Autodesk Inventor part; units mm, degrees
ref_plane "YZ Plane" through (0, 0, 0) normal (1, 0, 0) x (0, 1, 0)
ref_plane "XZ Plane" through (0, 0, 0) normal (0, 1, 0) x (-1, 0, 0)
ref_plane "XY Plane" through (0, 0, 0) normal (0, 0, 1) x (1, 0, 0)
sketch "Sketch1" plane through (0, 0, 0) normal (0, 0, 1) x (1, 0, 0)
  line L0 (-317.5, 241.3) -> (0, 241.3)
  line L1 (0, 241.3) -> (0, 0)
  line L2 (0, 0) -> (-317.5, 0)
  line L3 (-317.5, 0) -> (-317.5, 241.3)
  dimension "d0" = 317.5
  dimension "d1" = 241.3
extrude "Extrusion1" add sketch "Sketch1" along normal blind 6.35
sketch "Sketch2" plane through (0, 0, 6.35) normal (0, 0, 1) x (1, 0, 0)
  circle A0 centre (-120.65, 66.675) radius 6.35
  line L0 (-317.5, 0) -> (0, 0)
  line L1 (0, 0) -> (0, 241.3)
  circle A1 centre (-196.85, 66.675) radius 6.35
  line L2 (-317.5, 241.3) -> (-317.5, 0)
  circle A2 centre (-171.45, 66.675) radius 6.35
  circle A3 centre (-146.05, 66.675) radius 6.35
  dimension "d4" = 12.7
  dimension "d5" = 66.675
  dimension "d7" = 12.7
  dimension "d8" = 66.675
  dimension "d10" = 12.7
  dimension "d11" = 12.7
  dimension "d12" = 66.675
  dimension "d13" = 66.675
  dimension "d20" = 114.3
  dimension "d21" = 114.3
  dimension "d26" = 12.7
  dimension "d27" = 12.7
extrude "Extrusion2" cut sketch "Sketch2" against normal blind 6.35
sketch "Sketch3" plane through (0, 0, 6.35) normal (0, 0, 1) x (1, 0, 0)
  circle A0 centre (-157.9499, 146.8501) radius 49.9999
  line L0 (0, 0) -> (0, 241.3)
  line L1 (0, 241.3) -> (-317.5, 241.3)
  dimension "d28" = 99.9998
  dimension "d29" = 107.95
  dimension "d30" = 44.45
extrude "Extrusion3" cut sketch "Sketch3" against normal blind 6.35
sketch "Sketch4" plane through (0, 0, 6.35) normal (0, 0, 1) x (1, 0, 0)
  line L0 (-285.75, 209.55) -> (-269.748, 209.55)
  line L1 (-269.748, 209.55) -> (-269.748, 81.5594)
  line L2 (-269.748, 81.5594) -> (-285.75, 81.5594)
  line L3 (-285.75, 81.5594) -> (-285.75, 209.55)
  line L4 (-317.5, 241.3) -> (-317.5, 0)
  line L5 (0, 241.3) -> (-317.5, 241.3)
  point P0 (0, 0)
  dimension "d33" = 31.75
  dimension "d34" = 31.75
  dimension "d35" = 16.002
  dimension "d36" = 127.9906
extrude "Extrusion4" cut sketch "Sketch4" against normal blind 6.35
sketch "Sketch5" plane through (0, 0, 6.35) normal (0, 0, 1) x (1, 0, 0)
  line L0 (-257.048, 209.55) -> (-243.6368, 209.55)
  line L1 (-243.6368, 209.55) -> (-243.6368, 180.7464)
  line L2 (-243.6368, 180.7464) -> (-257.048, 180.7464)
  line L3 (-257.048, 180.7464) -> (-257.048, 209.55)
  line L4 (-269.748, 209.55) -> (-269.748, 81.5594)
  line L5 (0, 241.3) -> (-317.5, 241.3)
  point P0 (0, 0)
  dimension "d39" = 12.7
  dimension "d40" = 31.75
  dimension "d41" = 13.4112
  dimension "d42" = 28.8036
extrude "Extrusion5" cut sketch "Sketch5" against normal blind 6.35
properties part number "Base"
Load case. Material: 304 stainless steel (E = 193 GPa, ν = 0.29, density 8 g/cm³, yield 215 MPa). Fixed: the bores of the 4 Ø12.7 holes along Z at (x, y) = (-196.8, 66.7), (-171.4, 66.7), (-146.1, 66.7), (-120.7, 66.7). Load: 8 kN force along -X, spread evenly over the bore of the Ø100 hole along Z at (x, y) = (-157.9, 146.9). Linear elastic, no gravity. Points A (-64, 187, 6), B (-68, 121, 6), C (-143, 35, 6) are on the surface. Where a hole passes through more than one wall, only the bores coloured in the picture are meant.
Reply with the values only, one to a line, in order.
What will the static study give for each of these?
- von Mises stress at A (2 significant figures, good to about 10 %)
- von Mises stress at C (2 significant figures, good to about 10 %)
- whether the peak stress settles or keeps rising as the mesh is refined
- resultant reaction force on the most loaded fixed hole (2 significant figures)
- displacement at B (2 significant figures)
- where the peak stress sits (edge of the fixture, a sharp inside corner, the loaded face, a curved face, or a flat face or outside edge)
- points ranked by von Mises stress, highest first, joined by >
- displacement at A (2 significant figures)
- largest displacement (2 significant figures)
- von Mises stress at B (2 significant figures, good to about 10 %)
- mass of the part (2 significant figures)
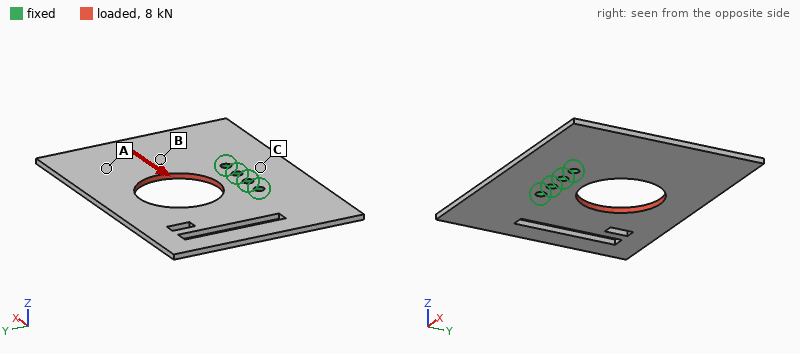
4.1 MPa
16 MPa
keeps rising
7.3 kN
25 µm
edge of the fixture
C > B > A
45 µm
67 µm
8.6 MPa
3.3 kg
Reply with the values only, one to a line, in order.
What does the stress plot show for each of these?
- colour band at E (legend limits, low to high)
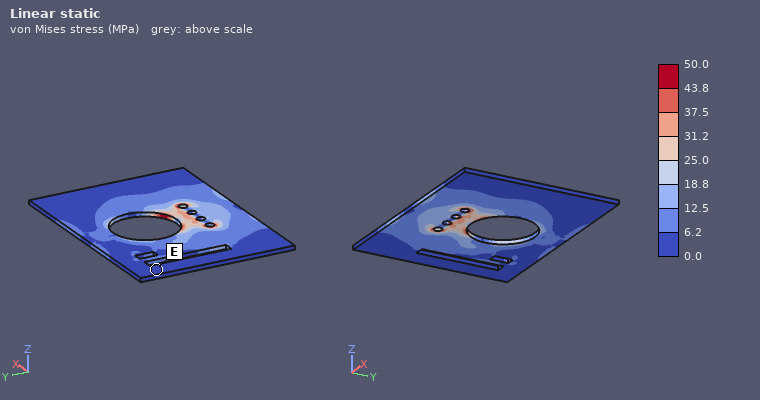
0.0 to 6.2 MPa
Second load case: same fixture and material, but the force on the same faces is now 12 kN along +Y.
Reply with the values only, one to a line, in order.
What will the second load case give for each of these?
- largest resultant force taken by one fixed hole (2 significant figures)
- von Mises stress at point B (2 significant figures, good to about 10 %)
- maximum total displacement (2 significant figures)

5.3 kN
6.2 MPa
18 µm
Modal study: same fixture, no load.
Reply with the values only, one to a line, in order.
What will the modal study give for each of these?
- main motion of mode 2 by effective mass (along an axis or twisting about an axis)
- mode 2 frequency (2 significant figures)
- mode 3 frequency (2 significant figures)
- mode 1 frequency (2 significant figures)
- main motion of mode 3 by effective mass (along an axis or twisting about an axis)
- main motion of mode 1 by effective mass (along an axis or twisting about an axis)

twisting about Y
170 Hz
300 Hz
120 Hz
along Z
along Z
